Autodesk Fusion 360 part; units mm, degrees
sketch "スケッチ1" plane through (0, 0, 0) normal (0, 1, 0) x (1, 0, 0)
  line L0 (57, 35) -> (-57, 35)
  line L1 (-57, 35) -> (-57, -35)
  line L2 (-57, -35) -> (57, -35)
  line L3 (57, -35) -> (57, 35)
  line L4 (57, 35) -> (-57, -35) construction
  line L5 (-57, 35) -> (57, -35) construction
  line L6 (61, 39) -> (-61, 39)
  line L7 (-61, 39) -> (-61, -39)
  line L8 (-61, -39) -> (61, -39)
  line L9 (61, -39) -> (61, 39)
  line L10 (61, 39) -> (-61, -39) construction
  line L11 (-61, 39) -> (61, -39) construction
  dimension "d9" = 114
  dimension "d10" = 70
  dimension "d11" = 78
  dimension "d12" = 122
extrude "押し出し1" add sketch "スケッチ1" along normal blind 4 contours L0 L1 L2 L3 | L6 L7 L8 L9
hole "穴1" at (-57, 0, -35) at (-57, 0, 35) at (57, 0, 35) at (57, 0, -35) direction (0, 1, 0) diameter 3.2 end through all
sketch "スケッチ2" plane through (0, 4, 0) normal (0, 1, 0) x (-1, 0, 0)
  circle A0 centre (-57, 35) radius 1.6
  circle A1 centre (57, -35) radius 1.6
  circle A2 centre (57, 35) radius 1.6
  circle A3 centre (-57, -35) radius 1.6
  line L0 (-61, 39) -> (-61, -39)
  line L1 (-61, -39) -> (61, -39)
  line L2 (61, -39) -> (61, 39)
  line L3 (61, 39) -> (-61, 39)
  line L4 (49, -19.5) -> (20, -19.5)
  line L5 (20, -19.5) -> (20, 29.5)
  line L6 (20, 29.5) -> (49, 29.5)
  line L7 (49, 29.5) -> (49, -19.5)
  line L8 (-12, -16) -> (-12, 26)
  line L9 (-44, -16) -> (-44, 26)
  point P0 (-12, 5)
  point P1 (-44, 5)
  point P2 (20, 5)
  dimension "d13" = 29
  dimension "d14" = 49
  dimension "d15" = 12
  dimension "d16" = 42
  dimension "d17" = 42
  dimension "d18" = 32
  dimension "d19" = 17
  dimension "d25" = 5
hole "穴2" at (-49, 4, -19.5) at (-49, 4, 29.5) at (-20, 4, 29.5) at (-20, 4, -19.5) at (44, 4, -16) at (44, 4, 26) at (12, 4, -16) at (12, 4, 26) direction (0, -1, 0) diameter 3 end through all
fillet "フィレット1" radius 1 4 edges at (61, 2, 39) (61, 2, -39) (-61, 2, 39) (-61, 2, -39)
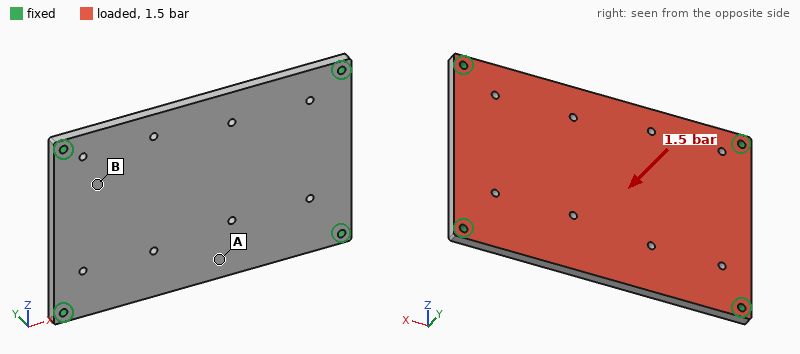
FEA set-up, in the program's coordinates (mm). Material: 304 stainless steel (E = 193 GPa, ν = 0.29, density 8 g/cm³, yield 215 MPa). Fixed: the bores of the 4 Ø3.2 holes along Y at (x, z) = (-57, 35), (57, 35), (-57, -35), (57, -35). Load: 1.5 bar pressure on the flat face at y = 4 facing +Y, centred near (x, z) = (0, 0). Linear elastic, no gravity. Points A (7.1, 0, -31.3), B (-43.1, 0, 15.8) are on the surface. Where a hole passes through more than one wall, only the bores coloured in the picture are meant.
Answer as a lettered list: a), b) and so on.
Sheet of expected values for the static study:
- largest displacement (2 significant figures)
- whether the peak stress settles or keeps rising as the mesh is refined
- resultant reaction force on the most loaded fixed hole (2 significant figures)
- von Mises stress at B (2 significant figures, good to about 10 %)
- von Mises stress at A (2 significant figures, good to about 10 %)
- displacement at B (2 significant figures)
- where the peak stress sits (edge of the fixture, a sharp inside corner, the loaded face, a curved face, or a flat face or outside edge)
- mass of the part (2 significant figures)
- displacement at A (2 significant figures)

a) 0.12 mm
b) keeps rising
c) 350 N
d) 16 MPa
e) 41 MPa
f) 0.043 mm
g) edge of the fixture
h) 300 g
i) 0.11 mm
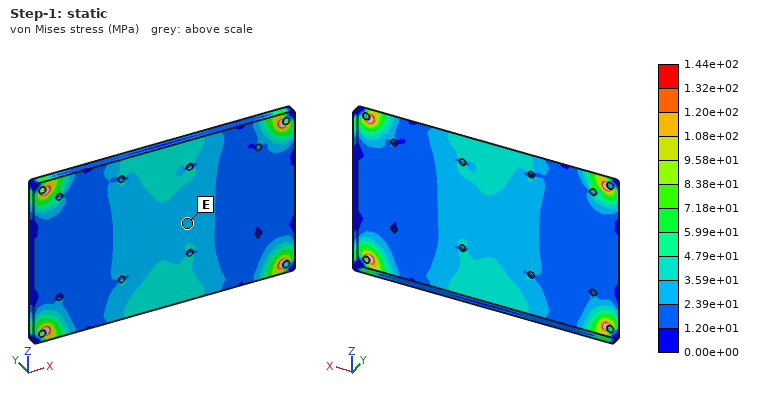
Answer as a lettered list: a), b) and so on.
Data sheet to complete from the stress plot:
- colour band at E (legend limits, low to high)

a) 2.39e+01 to 3.59e+01 MPa
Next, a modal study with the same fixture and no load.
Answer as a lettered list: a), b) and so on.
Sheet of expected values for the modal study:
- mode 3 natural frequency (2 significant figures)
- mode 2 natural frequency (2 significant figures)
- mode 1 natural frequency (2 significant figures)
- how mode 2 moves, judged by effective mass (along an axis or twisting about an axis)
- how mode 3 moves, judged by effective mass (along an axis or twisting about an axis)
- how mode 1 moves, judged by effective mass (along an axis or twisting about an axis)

a) 3000 Hz
b) 2100 Hz
c) 1200 Hz
d) twisting about X
e) twisting about Z
f) along Y
